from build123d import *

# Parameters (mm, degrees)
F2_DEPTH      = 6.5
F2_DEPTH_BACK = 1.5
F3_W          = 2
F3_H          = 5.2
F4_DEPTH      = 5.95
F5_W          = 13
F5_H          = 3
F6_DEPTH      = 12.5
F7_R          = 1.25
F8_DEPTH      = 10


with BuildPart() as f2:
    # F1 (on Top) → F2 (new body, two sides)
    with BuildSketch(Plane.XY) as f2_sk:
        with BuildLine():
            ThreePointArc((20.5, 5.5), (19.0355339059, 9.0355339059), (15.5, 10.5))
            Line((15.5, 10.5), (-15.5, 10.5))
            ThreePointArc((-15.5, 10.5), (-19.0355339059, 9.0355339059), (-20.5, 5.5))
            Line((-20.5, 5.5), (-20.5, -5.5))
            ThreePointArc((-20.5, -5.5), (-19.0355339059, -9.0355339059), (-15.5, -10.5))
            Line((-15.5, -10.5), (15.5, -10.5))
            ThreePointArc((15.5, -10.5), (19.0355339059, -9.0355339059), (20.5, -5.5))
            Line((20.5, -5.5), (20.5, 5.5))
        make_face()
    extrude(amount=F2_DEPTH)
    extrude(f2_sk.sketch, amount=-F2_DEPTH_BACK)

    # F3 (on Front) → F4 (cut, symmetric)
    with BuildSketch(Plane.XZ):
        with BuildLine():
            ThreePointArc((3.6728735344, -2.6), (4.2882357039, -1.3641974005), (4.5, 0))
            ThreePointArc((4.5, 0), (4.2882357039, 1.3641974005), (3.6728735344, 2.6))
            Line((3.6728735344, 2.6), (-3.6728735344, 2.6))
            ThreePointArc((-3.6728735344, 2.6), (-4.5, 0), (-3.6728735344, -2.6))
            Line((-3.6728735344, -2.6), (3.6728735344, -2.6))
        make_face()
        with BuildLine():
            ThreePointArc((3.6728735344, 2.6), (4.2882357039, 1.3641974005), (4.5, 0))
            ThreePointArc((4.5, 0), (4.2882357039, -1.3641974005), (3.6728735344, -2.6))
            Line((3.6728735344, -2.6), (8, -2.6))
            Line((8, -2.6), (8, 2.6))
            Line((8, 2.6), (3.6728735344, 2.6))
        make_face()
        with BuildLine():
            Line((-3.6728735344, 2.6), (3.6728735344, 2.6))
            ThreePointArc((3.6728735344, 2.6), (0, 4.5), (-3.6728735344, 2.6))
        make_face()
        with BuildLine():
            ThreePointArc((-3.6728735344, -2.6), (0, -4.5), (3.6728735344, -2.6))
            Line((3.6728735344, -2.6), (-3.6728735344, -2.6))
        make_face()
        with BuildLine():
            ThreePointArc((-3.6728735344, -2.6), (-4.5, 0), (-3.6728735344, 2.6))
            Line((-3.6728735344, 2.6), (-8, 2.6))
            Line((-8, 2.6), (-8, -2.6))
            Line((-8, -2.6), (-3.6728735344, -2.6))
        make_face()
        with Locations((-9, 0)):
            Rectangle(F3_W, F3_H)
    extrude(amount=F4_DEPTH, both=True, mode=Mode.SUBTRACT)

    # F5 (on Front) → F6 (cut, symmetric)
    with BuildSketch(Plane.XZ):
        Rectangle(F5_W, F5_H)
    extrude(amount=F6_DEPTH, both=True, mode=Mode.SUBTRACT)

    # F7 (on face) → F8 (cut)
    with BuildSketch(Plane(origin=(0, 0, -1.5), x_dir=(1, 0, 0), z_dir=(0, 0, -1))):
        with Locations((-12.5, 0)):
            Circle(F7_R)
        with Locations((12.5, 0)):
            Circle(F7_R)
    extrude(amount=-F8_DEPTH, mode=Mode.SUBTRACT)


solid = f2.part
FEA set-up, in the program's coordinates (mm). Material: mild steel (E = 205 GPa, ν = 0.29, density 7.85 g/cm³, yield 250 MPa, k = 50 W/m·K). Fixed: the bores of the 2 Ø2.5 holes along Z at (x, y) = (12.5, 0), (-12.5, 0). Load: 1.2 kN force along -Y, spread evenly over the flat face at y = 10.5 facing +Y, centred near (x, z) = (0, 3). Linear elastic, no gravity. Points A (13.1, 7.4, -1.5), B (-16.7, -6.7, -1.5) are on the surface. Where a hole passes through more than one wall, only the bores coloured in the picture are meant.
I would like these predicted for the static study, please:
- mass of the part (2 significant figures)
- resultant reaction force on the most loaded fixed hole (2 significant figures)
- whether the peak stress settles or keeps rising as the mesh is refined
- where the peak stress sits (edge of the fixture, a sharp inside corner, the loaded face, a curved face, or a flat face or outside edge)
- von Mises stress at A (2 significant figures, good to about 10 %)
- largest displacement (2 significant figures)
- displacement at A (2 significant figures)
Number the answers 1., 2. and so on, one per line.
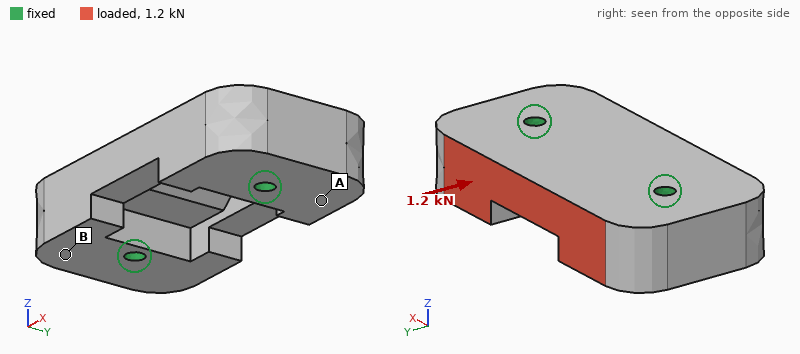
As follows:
1. 42 g
2. 610 N
3. keeps rising
4. edge of the fixture
5. 6.2 MPa
6. 1.0 µm
7. 0.26 µm
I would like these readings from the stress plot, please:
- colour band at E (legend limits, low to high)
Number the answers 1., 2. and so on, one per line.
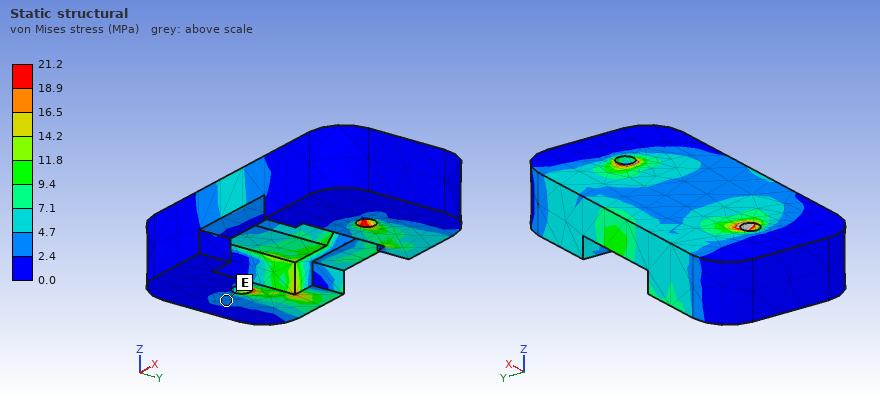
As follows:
1. 2.4 to 4.7 MPa
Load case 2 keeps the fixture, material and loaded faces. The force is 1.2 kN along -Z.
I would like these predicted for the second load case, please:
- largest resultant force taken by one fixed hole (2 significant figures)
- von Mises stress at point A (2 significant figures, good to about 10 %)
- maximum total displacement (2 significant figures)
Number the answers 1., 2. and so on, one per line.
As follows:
1. 640 N
2. 18 MPa
3. 7.5 µm
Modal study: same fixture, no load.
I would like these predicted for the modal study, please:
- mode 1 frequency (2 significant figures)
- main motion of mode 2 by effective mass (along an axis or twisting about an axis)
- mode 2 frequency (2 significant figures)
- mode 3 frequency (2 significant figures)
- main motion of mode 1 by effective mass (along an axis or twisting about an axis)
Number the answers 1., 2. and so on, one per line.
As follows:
1. 28 kHz
2. along Z
3. 30 kHz
4. 33 kHz
5. twisting about X
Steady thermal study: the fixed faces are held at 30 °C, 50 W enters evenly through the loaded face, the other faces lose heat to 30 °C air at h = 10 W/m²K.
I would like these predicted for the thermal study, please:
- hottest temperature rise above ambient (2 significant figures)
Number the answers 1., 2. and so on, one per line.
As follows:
1. 71 K
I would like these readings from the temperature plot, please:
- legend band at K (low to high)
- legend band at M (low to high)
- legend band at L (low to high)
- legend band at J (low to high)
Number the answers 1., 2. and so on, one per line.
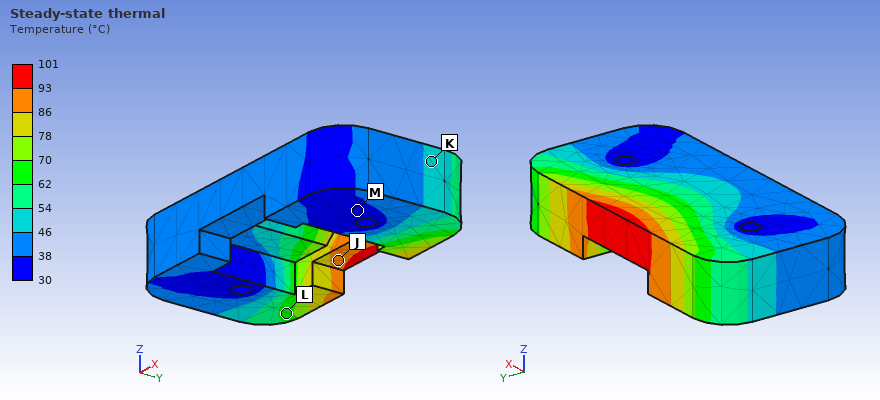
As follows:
1. 46 to 54 °C
2. 30 to 38 °C
3. 62 to 70 °C
4. 86 to 93 °C
